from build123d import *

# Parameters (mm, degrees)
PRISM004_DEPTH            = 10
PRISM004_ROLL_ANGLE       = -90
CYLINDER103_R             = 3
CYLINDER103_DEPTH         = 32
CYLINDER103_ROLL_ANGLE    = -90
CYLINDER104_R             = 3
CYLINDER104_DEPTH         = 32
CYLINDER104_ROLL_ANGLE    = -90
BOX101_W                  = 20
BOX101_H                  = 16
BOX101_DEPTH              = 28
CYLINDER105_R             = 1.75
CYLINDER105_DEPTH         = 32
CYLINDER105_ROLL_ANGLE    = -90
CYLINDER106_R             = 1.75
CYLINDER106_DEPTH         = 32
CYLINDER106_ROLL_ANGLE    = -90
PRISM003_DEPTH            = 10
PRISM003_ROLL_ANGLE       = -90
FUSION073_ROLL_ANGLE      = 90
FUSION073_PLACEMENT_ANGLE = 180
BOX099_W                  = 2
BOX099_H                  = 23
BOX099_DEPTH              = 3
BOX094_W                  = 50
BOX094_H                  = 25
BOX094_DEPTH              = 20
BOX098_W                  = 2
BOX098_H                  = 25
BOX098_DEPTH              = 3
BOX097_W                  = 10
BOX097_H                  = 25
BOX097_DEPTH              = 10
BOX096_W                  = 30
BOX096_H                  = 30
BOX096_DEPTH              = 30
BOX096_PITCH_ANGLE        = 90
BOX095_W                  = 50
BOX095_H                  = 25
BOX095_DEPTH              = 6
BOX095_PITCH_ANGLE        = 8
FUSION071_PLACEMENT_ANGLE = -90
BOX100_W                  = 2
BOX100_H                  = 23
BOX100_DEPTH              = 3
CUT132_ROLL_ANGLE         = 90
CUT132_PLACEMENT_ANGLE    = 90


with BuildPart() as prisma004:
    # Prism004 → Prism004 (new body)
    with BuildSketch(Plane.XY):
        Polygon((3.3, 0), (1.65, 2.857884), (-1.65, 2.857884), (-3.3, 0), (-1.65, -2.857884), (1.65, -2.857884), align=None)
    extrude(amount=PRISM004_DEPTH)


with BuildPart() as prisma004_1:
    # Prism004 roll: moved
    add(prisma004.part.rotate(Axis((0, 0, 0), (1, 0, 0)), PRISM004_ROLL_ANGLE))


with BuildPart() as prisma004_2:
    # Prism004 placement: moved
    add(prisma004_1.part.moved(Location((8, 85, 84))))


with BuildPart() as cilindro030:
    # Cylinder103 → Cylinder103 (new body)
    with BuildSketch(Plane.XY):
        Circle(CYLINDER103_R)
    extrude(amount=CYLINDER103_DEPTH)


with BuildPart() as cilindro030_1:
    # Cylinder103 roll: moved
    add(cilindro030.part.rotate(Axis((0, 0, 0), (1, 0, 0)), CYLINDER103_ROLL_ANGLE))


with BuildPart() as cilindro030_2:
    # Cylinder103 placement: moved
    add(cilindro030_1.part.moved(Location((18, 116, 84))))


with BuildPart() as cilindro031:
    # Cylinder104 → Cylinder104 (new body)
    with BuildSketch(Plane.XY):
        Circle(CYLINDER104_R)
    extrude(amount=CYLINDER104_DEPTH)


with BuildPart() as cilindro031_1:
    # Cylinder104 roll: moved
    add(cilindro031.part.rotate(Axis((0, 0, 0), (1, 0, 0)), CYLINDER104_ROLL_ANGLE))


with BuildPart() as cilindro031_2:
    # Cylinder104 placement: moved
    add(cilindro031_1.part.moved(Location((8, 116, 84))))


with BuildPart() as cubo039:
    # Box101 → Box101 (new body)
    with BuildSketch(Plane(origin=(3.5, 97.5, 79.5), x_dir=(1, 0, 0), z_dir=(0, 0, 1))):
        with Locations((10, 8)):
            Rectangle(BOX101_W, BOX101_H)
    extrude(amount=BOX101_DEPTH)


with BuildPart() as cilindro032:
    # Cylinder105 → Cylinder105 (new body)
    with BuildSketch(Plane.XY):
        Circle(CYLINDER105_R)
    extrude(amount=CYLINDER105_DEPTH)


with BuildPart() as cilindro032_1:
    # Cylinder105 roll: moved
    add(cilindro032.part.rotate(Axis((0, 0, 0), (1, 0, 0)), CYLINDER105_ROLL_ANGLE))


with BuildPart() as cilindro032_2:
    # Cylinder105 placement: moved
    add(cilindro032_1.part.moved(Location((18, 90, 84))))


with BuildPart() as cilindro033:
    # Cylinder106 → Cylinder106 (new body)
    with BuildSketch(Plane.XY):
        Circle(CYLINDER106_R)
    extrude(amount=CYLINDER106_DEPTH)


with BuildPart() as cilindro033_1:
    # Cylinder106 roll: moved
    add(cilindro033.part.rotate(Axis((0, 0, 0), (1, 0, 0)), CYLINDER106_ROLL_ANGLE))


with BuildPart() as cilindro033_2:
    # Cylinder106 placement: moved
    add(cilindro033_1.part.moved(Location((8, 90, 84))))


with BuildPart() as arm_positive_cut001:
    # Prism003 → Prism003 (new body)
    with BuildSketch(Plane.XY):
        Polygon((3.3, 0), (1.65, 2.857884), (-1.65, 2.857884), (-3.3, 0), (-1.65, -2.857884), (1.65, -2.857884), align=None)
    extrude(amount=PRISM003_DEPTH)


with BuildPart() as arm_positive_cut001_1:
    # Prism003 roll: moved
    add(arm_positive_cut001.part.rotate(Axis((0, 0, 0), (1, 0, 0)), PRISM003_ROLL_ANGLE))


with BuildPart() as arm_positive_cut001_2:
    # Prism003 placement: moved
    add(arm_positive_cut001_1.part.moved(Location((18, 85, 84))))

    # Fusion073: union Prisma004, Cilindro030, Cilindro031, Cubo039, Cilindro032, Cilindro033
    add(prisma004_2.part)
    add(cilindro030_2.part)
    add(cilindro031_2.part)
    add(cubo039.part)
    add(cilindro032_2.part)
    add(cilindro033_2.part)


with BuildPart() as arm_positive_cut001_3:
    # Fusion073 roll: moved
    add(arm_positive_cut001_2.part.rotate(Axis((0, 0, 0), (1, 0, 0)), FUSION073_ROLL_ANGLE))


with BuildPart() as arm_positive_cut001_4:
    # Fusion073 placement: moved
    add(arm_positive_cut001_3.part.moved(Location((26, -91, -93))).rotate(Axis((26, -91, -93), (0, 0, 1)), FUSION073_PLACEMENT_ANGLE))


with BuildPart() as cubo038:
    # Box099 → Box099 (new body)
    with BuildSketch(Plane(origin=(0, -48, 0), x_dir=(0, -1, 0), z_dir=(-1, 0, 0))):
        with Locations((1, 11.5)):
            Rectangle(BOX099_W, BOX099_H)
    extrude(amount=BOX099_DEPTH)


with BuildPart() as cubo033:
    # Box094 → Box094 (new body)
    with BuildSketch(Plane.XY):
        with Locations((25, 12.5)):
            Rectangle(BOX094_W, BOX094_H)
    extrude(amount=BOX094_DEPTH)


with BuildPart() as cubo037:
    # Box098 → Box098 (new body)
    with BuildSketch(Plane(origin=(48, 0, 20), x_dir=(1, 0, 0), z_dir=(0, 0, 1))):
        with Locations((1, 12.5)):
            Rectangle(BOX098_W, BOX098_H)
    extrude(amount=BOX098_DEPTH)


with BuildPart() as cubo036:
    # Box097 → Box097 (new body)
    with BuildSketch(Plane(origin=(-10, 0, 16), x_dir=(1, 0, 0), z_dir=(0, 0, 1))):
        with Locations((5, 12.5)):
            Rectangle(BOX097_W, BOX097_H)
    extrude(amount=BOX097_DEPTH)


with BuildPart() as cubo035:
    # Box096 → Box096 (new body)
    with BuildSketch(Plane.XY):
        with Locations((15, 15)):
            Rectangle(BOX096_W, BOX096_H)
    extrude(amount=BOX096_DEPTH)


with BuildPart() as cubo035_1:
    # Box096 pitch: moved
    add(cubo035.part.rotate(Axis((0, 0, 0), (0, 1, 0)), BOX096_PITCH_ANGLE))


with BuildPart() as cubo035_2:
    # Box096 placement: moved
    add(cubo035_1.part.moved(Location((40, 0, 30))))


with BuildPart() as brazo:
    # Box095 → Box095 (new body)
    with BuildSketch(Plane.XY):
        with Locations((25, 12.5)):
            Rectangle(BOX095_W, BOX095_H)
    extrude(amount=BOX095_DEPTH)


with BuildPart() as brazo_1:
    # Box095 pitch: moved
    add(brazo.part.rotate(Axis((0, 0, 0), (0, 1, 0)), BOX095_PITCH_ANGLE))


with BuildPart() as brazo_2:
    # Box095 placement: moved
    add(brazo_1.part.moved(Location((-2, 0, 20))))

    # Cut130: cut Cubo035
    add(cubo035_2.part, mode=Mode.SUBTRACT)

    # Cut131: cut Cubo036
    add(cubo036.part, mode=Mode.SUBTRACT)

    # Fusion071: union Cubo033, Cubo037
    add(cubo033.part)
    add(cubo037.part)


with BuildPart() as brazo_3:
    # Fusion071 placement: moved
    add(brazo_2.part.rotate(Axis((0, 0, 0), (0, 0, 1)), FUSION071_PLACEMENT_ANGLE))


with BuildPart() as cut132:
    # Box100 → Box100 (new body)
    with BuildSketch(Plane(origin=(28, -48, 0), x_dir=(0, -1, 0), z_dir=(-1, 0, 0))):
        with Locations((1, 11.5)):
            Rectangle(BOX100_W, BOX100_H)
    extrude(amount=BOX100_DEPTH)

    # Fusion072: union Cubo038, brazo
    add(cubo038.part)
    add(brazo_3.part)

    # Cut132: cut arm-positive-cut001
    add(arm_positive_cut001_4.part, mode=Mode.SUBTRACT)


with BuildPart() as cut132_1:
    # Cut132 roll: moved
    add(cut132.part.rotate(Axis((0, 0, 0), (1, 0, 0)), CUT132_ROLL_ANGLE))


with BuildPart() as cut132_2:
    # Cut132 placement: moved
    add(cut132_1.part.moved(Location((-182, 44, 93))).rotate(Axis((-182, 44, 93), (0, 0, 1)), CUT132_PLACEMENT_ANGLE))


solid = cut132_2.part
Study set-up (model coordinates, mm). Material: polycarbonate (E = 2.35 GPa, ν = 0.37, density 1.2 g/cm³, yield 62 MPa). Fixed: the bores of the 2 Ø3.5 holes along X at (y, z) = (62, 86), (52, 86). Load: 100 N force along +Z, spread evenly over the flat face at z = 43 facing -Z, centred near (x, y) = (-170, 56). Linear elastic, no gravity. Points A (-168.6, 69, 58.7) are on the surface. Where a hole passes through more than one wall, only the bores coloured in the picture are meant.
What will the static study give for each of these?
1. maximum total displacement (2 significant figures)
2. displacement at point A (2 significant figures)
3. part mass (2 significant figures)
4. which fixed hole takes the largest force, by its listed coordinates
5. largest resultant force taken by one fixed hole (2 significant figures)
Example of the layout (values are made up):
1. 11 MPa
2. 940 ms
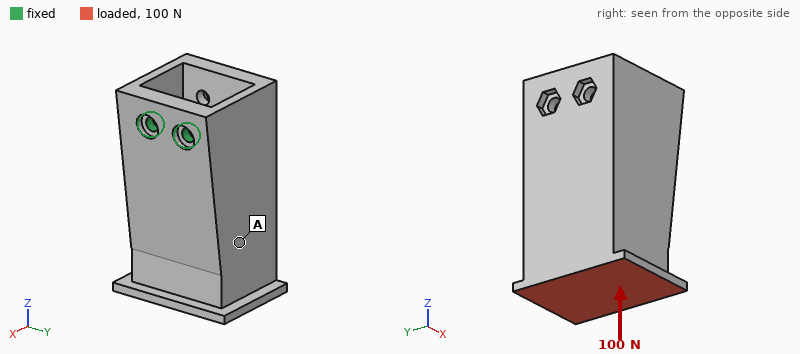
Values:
1. 0.72 mm
2. 0.42 mm
3. 29 g
4. (52, 86)
5. 58 N
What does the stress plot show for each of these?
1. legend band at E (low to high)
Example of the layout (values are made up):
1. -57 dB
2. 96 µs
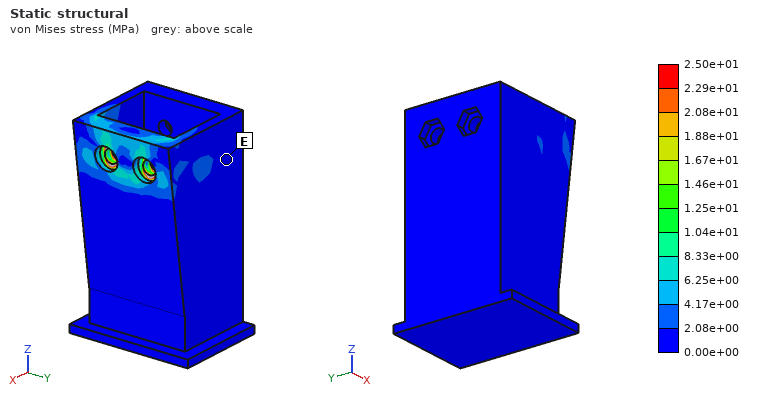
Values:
1. 0.00e+00 to 2.08e+00 MPa
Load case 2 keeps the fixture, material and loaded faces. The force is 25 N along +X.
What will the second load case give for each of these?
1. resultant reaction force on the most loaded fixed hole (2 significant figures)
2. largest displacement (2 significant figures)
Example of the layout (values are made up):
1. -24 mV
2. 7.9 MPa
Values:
1. 20 N
2. 0.74 mm
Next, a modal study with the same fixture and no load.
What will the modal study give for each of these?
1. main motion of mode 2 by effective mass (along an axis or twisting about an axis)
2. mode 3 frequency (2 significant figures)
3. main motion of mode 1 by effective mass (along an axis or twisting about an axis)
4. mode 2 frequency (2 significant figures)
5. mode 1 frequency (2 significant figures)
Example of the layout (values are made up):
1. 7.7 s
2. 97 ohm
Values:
1. along Y
2. 1400 Hz
3. along X
4. 850 Hz
5. 290 Hz
